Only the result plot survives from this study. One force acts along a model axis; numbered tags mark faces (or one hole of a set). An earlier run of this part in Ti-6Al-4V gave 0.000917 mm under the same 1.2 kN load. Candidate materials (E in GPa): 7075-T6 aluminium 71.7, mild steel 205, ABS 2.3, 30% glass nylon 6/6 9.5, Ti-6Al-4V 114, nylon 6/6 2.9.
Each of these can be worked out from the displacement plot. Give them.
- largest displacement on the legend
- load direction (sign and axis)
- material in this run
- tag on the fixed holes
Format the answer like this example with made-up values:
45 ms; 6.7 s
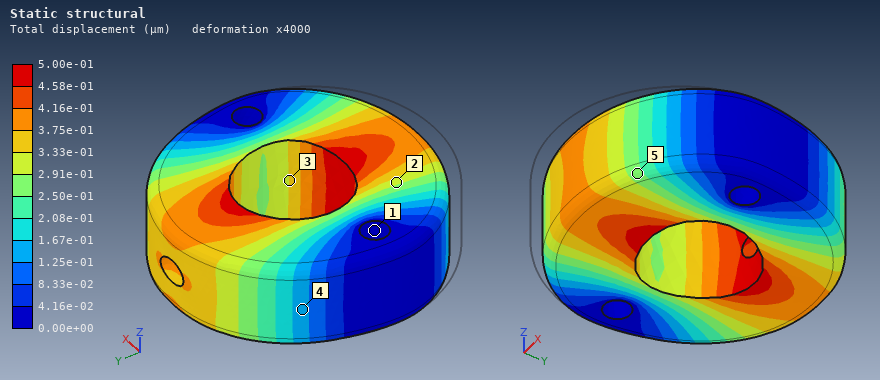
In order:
5.00e-01 µm; +Y; mild steel; 1
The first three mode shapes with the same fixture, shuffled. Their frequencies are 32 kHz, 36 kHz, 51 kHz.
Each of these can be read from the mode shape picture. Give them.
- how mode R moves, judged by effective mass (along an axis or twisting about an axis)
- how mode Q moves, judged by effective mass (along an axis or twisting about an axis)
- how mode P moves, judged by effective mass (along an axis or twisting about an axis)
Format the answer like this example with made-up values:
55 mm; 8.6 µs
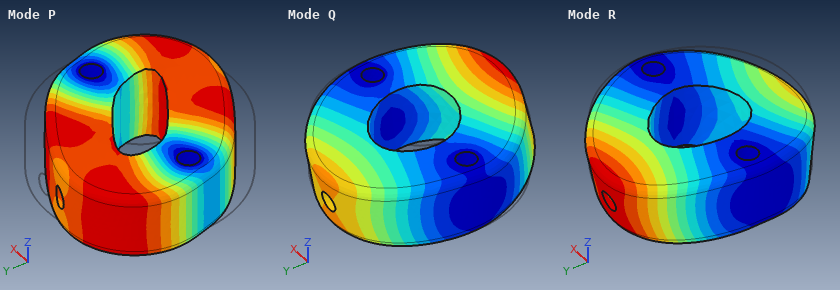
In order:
along Z; twisting about X; twisting about Z
